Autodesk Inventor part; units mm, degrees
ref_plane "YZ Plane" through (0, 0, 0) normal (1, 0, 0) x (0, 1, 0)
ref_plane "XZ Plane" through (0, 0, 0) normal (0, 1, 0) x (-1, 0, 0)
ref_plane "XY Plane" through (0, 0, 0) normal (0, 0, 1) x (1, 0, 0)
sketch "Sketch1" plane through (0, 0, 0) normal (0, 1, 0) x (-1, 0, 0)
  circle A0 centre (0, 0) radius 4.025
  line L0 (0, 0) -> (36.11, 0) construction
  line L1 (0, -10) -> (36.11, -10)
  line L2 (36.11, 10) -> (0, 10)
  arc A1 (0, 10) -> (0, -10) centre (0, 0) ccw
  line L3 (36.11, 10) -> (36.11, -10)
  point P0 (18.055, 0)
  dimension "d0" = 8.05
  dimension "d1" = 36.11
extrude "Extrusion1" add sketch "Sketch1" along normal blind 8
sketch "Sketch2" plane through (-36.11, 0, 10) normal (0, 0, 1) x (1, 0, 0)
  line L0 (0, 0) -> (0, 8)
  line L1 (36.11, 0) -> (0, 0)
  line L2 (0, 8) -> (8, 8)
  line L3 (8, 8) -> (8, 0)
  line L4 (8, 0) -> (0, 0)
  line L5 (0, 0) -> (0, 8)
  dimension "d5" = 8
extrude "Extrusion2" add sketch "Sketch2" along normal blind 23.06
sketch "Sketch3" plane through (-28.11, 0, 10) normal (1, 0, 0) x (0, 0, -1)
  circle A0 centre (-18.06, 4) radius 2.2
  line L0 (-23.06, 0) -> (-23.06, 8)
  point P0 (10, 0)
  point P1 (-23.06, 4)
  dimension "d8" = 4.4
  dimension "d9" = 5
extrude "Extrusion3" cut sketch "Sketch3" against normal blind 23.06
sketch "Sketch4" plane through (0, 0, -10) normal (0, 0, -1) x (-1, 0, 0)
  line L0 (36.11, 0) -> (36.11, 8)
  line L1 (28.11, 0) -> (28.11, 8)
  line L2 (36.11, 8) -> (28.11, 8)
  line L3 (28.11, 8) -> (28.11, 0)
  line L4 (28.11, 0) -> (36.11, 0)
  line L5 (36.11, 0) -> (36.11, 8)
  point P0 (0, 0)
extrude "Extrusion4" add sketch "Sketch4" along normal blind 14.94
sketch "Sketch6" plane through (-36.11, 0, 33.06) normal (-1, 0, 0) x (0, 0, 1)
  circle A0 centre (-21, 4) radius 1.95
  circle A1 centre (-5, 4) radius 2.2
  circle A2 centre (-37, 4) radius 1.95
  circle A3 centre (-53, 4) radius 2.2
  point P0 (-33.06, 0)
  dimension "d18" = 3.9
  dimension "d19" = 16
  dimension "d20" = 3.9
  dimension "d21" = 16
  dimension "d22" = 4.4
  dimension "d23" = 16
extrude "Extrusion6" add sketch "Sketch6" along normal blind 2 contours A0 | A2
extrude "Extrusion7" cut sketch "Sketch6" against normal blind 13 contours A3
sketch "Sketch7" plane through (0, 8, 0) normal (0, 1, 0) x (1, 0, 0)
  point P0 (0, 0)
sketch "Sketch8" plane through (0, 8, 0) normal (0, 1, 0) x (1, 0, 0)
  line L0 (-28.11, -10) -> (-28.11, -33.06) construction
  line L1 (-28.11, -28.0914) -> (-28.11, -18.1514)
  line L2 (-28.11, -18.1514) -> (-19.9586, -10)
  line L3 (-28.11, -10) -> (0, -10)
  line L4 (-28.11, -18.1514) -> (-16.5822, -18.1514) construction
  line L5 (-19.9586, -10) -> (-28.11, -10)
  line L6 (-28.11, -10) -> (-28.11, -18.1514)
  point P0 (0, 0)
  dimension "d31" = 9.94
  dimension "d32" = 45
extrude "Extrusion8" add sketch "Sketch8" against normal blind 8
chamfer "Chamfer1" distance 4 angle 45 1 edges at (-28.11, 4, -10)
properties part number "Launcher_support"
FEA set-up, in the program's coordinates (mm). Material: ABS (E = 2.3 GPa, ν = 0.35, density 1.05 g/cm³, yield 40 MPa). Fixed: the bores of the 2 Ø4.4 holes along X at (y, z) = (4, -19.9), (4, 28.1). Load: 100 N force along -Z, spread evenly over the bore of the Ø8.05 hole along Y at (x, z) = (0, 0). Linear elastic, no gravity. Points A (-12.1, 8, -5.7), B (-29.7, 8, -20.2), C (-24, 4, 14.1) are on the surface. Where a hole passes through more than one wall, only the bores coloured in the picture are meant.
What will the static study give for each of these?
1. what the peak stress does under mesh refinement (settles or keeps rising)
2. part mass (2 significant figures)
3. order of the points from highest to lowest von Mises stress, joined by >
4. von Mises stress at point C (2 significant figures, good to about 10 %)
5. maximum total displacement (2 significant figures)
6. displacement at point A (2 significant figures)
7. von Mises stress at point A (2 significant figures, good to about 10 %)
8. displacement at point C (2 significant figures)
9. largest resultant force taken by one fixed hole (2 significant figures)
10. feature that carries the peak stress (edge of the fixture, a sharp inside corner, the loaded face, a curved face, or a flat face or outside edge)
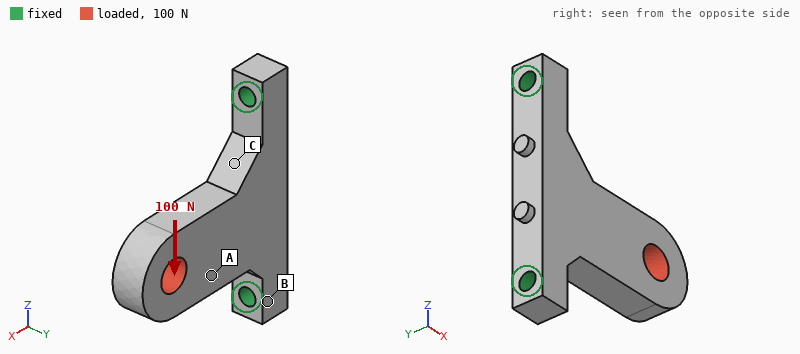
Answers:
keeps rising
9.7 g
C > A > B
4.4 MPa
0.18 mm
0.066 mm
1.5 MPa
0.034 mm
100 N
edge of the fixture
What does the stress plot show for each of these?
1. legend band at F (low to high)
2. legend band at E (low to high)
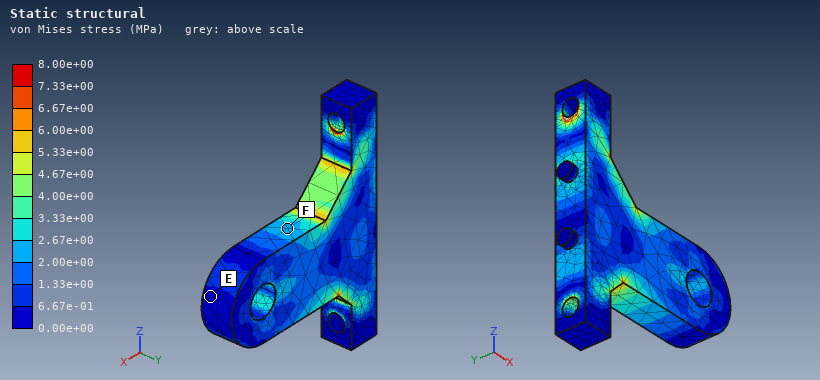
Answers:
2.00e+00 to 2.67e+00 MPa
0.00e+00 to 6.67e-01 MPa
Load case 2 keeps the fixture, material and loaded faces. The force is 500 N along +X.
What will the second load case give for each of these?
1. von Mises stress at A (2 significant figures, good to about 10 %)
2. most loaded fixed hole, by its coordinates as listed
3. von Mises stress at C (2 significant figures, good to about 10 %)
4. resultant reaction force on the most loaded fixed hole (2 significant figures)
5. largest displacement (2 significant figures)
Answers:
3.2 MPa
(4, -19.9)
8.7 MPa
330 N
0.17 mm
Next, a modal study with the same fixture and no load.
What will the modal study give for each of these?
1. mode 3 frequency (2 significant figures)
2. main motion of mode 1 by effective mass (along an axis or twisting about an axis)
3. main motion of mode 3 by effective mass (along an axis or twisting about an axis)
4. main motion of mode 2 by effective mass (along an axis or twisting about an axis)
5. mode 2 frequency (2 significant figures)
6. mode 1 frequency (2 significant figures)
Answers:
3500 Hz
along Y
along Y
along Z
2500 Hz
730 Hz
